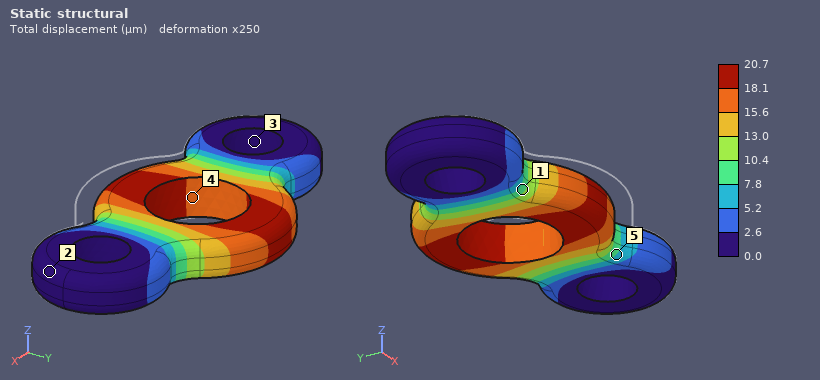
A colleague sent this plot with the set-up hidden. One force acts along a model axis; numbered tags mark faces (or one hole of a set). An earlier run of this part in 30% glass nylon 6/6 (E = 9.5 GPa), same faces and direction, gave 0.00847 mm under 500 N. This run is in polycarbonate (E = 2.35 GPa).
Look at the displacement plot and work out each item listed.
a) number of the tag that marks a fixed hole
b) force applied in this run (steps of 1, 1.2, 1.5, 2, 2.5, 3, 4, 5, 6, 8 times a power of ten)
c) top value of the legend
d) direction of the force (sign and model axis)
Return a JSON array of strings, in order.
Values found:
["3", "300 N", "20.7 µm", "+Y"]
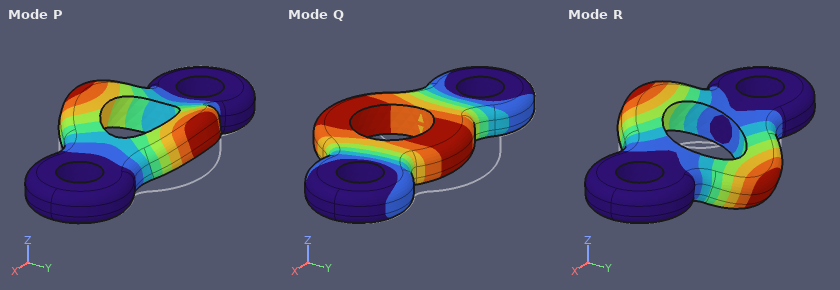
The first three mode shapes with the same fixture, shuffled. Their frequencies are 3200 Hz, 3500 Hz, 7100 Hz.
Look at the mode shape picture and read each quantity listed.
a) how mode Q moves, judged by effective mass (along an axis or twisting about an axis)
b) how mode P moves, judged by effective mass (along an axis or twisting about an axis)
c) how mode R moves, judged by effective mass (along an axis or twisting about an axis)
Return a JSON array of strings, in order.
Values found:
["along Y", "along Z", "twisting about X"]
